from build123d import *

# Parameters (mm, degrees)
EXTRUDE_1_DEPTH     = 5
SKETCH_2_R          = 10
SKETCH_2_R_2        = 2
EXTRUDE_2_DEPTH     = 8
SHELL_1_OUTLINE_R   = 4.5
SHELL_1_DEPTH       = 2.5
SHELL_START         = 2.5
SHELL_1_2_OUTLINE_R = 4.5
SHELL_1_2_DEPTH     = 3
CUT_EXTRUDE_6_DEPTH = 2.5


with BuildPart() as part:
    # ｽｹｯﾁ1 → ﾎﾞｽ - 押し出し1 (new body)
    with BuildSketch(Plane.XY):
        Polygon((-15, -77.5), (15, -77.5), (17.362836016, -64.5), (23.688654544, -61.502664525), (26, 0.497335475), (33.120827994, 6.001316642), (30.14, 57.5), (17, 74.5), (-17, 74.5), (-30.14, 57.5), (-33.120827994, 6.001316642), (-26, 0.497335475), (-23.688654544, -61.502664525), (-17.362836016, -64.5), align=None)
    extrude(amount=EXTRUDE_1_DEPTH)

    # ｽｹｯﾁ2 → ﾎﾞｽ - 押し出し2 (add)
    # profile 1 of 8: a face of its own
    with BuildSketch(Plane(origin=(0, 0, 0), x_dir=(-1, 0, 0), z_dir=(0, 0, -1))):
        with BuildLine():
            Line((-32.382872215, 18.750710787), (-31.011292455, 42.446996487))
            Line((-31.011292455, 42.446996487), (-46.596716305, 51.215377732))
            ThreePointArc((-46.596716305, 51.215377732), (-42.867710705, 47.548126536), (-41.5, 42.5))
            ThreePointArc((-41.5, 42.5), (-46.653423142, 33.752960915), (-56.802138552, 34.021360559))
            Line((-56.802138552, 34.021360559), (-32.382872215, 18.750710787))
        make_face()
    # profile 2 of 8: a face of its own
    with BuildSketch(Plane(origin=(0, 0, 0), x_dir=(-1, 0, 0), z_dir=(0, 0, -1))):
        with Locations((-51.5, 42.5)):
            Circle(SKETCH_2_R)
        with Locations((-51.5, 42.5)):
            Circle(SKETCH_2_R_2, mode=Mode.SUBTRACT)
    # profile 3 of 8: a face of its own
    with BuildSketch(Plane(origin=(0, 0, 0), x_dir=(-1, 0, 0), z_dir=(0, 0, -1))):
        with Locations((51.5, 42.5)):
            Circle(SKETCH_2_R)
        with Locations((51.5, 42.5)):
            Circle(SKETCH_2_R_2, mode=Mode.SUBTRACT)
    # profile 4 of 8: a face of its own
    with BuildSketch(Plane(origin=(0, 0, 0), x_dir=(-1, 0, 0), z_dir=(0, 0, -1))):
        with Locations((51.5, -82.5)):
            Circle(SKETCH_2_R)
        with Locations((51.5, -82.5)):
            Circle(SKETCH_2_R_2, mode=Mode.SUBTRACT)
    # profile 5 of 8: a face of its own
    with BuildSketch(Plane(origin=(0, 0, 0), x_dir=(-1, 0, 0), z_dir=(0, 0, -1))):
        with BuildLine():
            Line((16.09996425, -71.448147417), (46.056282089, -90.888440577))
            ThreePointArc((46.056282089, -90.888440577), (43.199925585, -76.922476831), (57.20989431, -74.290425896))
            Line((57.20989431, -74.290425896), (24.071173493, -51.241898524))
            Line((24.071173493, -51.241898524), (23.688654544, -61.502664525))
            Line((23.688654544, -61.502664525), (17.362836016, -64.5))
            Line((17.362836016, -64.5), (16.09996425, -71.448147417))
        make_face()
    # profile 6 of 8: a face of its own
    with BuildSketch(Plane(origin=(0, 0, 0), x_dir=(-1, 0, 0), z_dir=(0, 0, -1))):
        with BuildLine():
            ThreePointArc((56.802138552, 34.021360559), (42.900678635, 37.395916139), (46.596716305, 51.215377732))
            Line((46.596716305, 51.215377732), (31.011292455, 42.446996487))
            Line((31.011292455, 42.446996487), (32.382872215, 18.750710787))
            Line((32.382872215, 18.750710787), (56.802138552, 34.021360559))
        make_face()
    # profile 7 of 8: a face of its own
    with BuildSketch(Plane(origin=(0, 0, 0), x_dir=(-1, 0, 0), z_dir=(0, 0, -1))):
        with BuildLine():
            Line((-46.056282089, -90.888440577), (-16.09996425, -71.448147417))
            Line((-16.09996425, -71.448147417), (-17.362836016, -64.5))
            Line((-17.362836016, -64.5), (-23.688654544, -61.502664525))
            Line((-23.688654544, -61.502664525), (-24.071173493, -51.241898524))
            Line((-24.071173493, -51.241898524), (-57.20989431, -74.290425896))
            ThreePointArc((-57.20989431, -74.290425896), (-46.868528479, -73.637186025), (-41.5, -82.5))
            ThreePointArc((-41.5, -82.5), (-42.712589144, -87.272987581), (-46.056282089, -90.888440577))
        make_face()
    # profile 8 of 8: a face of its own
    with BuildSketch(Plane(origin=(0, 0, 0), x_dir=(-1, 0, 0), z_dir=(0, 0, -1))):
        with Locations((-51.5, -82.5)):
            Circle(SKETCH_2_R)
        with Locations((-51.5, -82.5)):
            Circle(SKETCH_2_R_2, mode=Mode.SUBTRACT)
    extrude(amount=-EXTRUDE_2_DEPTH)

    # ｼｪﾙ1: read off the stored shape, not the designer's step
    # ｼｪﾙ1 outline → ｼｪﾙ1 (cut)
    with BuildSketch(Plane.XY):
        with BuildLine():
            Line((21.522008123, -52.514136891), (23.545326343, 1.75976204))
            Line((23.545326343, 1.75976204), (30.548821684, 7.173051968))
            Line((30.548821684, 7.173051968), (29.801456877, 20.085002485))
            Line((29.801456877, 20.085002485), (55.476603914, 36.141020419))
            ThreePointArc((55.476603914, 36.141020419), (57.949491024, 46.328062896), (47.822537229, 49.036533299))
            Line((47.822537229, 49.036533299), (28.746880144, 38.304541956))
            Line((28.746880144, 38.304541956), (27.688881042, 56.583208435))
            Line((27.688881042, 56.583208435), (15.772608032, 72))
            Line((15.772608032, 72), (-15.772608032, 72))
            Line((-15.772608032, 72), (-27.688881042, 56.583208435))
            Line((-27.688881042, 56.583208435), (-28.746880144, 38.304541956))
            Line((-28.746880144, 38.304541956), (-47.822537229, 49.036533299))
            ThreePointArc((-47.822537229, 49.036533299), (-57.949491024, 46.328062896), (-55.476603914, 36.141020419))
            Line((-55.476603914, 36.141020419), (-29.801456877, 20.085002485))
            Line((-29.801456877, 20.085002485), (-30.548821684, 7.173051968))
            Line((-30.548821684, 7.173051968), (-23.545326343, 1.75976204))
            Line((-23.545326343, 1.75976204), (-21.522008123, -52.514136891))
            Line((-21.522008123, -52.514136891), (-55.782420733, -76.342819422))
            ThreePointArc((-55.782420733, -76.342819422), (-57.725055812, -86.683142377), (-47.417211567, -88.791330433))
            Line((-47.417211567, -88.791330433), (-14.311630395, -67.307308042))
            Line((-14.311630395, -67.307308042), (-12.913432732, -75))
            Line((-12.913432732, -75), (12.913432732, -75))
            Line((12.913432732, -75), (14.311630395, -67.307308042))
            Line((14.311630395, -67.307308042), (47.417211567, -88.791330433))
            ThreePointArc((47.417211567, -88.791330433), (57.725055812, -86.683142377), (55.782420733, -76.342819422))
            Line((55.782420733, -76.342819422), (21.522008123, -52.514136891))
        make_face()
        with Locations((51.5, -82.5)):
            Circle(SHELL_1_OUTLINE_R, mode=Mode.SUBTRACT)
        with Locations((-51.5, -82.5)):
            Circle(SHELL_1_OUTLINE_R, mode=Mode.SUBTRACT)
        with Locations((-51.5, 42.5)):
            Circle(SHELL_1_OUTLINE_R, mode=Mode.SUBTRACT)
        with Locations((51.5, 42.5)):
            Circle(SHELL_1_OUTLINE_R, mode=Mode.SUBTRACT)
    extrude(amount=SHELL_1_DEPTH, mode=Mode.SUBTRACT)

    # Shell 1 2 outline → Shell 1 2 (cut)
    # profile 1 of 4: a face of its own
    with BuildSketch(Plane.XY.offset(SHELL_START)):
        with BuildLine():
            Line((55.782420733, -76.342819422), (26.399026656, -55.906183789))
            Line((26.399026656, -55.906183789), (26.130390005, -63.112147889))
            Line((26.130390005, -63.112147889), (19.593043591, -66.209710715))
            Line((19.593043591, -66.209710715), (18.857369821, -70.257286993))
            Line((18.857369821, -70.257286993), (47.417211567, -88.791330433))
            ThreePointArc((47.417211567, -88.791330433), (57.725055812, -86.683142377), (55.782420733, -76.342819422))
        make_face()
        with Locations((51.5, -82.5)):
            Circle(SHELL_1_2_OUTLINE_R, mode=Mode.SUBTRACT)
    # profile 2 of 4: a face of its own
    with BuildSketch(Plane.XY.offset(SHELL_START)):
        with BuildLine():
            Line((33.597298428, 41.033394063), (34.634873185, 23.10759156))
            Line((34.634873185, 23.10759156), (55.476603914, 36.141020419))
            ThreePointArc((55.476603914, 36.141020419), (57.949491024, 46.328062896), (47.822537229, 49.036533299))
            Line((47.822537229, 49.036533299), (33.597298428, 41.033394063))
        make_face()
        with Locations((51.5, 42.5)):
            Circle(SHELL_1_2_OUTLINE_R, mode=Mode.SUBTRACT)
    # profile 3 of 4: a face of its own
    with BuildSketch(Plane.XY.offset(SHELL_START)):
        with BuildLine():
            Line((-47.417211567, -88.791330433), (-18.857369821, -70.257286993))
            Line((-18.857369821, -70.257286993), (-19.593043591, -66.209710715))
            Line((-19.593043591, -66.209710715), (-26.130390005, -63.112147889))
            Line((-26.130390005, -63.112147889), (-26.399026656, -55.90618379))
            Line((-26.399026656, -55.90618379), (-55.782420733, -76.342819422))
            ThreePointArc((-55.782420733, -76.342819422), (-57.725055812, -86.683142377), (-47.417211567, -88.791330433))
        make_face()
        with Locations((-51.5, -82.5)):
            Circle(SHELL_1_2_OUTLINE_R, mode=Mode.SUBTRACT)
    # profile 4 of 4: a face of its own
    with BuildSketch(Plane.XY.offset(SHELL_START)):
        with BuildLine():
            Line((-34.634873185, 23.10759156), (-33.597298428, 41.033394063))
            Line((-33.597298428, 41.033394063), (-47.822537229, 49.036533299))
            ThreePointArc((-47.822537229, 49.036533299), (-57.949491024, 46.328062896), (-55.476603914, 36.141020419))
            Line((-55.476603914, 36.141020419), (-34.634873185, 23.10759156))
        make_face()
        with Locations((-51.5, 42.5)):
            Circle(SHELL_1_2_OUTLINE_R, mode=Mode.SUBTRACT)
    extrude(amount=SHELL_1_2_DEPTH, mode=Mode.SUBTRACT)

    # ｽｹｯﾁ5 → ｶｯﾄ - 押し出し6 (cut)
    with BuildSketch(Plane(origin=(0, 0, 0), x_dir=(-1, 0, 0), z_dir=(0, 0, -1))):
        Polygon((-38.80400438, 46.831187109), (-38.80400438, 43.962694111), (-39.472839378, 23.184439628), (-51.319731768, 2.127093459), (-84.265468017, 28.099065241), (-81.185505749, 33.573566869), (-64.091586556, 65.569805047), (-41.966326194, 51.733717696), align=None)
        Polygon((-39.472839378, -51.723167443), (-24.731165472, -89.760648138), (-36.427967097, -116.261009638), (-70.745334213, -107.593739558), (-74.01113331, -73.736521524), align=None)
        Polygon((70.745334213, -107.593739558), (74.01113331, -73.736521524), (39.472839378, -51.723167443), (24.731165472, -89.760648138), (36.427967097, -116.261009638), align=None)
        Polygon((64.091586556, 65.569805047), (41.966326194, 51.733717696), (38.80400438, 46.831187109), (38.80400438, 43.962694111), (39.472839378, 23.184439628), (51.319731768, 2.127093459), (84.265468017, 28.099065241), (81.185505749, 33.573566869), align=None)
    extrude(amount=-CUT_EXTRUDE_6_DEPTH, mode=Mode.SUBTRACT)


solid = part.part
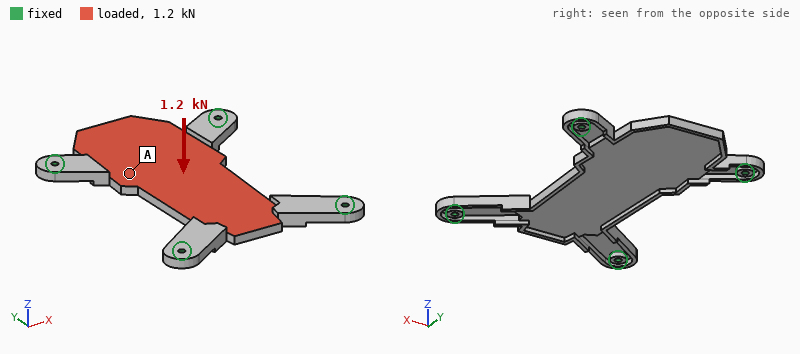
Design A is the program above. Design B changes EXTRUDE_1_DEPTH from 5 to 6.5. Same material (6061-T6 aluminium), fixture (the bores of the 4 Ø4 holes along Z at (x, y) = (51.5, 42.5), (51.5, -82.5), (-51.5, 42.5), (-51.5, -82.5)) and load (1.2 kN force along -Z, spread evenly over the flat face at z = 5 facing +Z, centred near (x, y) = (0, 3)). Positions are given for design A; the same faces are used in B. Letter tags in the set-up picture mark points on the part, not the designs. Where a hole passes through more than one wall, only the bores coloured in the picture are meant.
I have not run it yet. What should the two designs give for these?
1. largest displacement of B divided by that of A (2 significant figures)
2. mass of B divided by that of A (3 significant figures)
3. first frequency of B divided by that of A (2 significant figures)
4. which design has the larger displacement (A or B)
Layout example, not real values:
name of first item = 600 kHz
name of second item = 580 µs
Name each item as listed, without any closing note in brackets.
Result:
largest displacement of B divided by that of A = 0.67
mass of B divided by that of A = 1.35
first frequency of B divided by that of A = 0.96
which design has the larger displacement = A
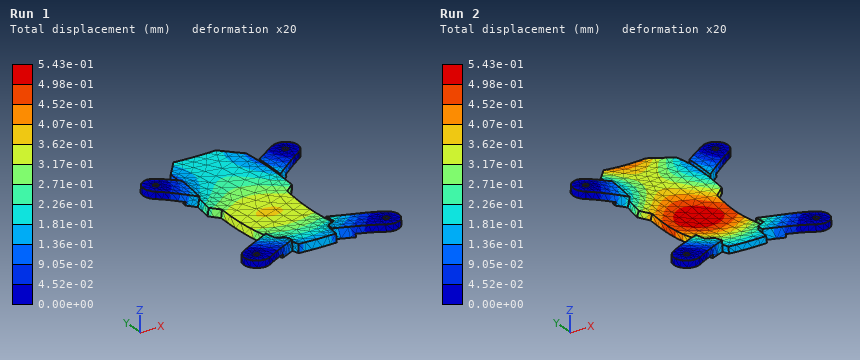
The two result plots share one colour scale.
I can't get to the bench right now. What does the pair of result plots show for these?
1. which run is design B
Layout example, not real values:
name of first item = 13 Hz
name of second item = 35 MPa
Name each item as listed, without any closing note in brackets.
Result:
which run is design B = Run 1
